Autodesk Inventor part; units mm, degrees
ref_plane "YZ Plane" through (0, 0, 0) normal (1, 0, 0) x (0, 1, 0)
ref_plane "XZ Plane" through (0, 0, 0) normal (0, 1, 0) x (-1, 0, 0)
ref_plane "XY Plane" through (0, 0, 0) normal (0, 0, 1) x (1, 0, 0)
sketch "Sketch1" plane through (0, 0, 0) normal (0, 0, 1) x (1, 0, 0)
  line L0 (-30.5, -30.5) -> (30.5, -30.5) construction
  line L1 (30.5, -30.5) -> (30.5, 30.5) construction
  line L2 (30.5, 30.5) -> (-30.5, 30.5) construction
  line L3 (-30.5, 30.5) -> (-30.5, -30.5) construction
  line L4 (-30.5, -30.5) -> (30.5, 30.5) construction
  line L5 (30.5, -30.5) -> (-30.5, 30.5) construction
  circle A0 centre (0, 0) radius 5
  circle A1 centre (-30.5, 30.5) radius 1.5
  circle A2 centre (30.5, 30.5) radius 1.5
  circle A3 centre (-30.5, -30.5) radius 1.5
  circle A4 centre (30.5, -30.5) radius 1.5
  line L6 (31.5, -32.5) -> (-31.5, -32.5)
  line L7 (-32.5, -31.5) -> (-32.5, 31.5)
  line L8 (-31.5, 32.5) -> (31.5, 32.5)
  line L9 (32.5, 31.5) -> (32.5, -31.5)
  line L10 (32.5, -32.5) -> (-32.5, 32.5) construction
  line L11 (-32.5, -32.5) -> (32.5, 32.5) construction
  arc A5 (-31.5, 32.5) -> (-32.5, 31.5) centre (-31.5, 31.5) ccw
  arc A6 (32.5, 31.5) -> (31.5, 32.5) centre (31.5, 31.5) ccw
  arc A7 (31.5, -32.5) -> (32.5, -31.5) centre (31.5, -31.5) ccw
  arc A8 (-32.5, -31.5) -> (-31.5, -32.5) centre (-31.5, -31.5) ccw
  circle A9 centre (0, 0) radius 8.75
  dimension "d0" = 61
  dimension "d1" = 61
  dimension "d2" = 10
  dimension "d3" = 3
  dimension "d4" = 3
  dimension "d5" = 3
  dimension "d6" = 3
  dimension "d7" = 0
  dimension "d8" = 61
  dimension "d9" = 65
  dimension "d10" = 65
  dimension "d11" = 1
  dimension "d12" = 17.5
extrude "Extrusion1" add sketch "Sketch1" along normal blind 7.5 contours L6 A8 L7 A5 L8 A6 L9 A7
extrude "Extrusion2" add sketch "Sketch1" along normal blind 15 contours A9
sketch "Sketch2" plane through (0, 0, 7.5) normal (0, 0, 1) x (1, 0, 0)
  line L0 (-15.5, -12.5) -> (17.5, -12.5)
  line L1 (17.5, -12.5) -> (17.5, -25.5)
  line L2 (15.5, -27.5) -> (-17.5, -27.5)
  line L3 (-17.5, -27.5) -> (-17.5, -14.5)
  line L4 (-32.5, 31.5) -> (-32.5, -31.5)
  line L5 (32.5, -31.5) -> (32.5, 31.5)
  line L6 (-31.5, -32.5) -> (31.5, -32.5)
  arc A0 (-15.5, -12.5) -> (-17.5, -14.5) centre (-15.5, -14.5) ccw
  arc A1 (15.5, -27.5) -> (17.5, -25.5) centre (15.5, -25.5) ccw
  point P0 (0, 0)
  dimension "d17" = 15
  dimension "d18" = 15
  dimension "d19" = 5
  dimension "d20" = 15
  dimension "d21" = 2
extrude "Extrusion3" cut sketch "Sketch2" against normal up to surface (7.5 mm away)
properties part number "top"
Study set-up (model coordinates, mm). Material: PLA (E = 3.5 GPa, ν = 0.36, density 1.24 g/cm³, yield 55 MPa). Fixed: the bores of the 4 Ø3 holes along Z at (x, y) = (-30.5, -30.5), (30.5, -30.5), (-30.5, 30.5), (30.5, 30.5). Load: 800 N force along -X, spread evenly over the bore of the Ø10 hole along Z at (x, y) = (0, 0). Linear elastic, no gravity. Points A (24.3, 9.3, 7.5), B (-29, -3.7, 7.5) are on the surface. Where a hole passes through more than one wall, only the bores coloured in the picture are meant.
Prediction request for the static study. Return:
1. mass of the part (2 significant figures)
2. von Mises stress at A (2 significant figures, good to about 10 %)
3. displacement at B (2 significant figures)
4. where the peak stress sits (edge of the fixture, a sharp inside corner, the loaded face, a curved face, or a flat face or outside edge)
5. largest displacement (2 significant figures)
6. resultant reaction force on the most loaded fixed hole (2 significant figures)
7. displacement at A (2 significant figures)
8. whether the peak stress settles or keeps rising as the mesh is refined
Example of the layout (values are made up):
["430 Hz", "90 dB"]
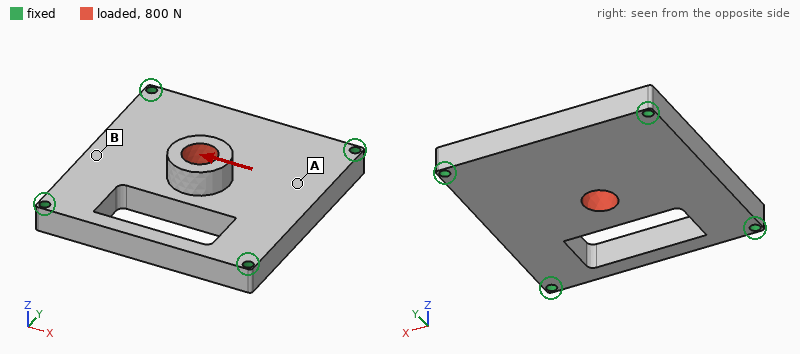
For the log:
["35 g", "2.5 MPa", "0.058 mm", "edge of the fixture", "0.10 mm", "390 N", "0.046 mm", "keeps rising"]
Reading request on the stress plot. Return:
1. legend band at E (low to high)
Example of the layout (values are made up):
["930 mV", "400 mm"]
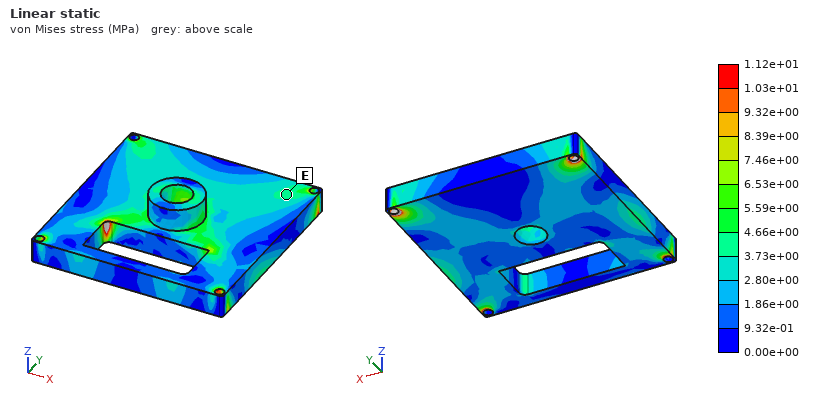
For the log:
["3.73e+00 to 4.66e+00 MPa"]
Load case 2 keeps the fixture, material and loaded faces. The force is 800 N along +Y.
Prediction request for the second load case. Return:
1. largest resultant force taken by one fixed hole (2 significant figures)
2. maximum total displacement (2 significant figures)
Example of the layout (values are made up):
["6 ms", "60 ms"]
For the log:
["270 N", "0.13 mm"]
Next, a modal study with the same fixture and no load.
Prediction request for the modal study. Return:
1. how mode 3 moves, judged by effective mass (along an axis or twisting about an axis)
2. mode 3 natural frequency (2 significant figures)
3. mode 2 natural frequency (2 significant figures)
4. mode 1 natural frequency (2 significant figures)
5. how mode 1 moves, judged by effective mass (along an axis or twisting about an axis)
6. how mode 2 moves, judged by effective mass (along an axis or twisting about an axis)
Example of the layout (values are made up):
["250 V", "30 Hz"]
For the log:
["twisting about X", "3300 Hz", "3000 Hz", "1700 Hz", "along Z", "twisting about Y"]
